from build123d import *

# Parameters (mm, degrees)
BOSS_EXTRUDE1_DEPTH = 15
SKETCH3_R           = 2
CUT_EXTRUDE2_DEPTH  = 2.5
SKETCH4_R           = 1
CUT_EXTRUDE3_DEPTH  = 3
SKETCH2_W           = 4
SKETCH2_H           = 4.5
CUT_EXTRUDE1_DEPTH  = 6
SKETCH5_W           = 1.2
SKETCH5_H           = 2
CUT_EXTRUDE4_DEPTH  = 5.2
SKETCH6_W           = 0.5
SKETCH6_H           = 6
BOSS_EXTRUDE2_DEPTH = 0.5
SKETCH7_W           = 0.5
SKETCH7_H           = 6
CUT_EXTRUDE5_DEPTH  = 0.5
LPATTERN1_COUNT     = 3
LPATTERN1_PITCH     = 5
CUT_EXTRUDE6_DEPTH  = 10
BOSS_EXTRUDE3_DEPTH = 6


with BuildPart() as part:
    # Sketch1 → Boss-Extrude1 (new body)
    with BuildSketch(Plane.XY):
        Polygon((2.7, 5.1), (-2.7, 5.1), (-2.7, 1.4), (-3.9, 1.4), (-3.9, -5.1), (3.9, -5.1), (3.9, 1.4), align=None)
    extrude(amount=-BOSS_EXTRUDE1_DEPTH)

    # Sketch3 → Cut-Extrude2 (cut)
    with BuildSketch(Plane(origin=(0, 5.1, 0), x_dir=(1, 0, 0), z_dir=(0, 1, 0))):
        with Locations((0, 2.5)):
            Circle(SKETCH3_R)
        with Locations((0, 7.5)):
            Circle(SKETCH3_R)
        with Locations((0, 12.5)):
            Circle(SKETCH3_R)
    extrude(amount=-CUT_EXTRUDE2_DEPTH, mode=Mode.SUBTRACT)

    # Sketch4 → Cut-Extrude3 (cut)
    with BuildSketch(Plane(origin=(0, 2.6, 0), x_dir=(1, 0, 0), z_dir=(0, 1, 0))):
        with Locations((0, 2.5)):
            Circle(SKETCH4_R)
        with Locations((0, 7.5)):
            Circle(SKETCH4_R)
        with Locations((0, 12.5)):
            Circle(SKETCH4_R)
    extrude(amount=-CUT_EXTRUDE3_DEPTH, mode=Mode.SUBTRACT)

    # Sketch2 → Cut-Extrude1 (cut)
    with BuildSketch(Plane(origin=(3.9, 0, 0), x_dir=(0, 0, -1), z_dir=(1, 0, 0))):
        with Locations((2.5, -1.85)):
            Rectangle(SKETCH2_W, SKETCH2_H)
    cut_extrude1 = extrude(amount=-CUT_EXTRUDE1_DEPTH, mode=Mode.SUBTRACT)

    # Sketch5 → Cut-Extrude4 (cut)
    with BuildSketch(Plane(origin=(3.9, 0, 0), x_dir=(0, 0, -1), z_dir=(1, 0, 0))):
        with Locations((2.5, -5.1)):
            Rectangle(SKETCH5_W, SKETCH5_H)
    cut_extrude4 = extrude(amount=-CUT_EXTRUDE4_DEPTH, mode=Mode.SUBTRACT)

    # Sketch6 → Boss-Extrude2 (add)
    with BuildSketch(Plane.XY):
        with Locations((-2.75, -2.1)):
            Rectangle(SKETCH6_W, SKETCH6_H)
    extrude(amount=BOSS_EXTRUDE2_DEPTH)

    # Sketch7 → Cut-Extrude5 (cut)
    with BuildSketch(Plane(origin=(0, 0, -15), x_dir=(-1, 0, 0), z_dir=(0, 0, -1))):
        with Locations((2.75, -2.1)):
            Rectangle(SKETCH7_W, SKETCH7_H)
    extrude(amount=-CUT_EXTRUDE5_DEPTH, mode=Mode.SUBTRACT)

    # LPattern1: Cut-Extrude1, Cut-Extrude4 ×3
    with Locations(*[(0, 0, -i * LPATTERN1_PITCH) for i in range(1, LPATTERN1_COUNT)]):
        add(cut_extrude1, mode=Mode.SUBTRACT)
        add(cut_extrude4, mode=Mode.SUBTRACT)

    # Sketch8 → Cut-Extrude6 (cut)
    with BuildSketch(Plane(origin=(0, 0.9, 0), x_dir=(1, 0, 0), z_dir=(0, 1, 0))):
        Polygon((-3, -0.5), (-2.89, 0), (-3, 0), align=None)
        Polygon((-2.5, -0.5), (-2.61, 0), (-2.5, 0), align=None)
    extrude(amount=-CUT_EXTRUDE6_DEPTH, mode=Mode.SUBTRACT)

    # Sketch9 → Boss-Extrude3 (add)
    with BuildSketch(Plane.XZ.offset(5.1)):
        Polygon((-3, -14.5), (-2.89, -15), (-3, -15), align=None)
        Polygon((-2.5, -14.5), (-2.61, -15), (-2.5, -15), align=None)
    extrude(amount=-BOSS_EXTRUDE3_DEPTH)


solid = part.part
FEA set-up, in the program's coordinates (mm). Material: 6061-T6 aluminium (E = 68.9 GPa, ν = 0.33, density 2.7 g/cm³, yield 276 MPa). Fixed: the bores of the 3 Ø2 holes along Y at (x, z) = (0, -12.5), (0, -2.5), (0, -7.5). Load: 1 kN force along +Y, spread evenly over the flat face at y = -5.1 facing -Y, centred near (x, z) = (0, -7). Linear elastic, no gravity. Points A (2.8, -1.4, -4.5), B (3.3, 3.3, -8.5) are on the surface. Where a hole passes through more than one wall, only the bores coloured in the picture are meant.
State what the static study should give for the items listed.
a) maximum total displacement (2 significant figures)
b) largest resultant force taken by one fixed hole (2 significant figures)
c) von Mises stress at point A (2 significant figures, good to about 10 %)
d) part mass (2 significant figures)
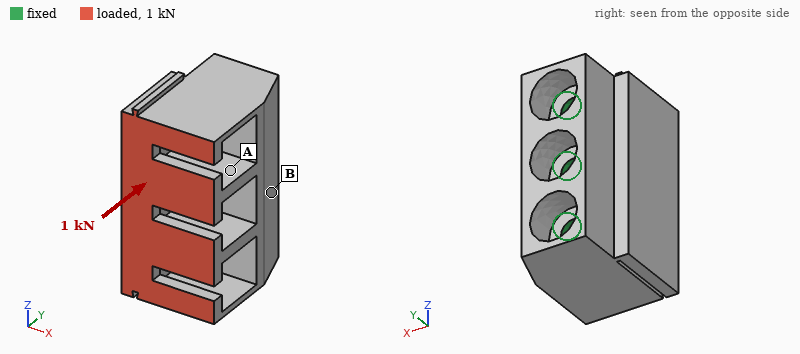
25 µm
340 N
37 MPa
1.7 g
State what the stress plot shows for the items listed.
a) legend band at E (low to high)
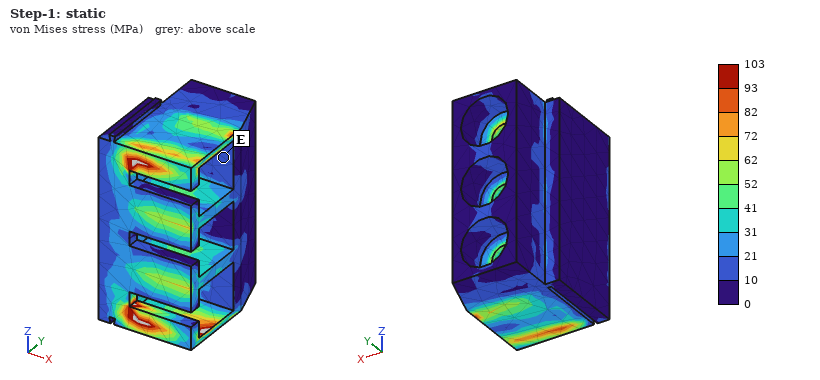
10 to 21 MPa
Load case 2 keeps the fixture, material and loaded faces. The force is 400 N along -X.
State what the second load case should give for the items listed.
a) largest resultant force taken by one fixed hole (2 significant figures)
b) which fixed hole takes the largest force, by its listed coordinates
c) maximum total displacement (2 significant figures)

150 N
(0, -7.5)
22 µm
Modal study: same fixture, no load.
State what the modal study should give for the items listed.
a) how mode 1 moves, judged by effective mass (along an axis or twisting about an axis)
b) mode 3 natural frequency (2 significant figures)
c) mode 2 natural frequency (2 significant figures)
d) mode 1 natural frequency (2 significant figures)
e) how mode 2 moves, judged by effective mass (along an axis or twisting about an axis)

along Z
37 kHz
35 kHz
32 kHz
along X
